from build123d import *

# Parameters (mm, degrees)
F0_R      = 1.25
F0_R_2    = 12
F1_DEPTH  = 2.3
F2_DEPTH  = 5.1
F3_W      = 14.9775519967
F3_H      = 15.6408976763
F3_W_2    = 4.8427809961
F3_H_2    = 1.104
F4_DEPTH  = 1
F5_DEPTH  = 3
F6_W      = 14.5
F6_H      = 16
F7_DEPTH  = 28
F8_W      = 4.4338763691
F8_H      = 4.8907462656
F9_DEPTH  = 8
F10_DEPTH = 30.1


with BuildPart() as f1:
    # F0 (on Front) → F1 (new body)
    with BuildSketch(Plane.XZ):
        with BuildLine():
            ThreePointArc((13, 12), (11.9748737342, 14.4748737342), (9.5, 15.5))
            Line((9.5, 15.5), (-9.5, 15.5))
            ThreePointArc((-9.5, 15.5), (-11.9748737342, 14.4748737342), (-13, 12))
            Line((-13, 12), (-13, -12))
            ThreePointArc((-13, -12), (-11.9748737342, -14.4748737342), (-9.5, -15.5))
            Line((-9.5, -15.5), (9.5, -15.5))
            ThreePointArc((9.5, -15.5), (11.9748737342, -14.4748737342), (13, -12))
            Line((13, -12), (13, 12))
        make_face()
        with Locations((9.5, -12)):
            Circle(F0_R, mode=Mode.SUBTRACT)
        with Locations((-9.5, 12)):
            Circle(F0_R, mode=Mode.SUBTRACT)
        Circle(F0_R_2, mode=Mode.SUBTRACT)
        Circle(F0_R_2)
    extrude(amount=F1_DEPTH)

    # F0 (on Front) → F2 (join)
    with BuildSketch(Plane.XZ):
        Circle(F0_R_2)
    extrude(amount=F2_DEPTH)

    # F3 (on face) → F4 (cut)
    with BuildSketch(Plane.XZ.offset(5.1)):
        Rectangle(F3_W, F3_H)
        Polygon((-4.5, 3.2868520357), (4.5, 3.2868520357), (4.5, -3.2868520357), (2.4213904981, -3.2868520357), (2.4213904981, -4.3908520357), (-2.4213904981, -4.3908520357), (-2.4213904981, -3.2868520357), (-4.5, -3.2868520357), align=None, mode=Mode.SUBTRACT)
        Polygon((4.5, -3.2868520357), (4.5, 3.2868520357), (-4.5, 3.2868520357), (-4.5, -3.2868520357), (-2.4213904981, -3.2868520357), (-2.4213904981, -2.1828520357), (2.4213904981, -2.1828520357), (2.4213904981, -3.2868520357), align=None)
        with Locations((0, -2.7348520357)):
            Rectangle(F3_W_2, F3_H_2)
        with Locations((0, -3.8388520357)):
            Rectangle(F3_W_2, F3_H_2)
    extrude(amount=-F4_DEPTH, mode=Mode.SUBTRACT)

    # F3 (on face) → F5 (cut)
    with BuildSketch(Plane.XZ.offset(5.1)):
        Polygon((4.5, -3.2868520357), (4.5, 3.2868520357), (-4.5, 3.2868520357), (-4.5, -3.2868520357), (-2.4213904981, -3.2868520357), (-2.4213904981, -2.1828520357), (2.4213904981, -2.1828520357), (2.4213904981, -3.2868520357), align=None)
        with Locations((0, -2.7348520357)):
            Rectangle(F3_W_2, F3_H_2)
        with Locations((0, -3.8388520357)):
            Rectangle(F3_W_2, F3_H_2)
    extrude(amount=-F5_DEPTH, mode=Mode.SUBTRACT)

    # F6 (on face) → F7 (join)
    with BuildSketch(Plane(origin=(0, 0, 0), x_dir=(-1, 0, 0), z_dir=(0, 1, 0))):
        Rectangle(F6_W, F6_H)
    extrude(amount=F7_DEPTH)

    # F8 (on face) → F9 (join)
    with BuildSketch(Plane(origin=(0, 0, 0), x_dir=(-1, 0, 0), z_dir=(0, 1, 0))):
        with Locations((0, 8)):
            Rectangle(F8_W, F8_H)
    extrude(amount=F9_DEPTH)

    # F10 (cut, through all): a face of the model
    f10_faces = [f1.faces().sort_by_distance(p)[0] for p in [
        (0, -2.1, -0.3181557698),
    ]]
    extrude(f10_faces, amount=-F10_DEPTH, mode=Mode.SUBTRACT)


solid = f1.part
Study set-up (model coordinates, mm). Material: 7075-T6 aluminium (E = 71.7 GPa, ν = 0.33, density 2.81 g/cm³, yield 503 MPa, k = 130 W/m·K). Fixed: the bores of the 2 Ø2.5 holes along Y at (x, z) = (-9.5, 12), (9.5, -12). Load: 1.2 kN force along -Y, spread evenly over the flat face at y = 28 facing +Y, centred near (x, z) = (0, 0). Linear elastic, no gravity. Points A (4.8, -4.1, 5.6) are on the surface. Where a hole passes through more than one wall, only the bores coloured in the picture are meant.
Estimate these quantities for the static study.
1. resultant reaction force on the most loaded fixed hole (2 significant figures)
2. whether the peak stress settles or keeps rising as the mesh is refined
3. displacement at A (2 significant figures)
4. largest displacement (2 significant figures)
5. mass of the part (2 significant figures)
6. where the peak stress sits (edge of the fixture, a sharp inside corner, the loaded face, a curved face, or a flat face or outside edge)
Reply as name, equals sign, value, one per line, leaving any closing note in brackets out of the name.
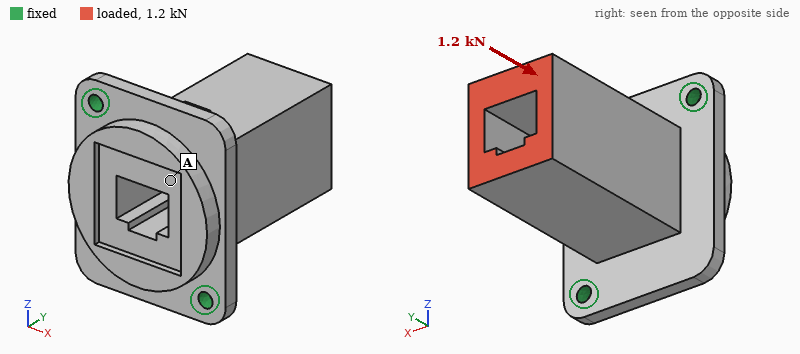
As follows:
resultant reaction force on the most loaded fixed hole = 600 N
whether the peak stress settles or keeps rising as the mesh is refined = keeps rising
displacement at A = 21 µm
largest displacement = 26 µm
mass of the part = 21 g
where the peak stress sits = edge of the fixture
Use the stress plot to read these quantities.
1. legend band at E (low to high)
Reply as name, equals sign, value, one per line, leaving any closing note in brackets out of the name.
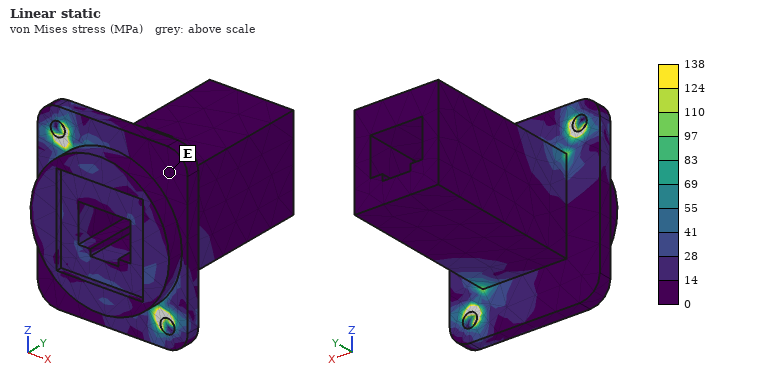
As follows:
legend band at E = 0 to 14 MPa
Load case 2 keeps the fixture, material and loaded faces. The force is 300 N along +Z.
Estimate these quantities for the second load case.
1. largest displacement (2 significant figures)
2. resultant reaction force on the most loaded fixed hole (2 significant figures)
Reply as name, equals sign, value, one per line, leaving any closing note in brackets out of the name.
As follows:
largest displacement = 0.27 mm
resultant reaction force on the most loaded fixed hole = 310 N
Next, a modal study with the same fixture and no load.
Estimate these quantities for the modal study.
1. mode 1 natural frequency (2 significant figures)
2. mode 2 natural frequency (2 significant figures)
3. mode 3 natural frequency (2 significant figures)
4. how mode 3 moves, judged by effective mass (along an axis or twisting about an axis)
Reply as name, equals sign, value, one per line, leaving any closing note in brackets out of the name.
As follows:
mode 1 natural frequency = 1800 Hz
mode 2 natural frequency = 6900 Hz
mode 3 natural frequency = 8700 Hz
how mode 3 moves, judged by effective mass = along Y
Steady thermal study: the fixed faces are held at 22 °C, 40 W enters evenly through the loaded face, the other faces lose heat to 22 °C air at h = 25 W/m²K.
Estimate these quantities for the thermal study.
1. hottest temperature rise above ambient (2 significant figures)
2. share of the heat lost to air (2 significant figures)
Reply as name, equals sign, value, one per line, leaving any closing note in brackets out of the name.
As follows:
hottest temperature rise above ambient = 82 K
share of the heat lost to air = 13 %
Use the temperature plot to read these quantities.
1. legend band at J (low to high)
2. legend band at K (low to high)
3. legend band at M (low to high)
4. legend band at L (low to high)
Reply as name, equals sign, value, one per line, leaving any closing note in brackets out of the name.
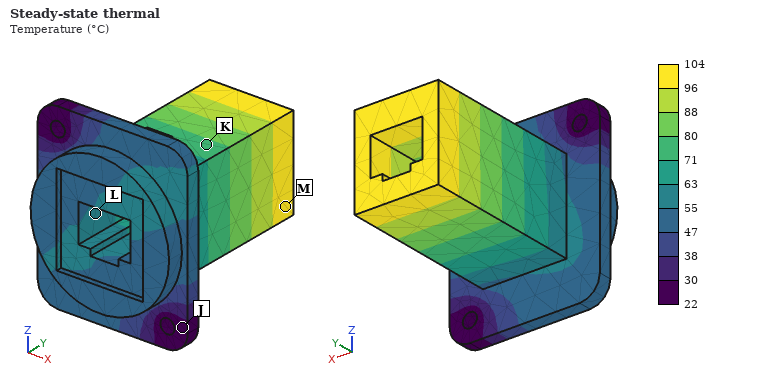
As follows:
legend band at J = 22 to 30 °C
legend band at K = 71 to 80 °C
legend band at M = 96 to 104 °C
legend band at L = 55 to 63 °C
